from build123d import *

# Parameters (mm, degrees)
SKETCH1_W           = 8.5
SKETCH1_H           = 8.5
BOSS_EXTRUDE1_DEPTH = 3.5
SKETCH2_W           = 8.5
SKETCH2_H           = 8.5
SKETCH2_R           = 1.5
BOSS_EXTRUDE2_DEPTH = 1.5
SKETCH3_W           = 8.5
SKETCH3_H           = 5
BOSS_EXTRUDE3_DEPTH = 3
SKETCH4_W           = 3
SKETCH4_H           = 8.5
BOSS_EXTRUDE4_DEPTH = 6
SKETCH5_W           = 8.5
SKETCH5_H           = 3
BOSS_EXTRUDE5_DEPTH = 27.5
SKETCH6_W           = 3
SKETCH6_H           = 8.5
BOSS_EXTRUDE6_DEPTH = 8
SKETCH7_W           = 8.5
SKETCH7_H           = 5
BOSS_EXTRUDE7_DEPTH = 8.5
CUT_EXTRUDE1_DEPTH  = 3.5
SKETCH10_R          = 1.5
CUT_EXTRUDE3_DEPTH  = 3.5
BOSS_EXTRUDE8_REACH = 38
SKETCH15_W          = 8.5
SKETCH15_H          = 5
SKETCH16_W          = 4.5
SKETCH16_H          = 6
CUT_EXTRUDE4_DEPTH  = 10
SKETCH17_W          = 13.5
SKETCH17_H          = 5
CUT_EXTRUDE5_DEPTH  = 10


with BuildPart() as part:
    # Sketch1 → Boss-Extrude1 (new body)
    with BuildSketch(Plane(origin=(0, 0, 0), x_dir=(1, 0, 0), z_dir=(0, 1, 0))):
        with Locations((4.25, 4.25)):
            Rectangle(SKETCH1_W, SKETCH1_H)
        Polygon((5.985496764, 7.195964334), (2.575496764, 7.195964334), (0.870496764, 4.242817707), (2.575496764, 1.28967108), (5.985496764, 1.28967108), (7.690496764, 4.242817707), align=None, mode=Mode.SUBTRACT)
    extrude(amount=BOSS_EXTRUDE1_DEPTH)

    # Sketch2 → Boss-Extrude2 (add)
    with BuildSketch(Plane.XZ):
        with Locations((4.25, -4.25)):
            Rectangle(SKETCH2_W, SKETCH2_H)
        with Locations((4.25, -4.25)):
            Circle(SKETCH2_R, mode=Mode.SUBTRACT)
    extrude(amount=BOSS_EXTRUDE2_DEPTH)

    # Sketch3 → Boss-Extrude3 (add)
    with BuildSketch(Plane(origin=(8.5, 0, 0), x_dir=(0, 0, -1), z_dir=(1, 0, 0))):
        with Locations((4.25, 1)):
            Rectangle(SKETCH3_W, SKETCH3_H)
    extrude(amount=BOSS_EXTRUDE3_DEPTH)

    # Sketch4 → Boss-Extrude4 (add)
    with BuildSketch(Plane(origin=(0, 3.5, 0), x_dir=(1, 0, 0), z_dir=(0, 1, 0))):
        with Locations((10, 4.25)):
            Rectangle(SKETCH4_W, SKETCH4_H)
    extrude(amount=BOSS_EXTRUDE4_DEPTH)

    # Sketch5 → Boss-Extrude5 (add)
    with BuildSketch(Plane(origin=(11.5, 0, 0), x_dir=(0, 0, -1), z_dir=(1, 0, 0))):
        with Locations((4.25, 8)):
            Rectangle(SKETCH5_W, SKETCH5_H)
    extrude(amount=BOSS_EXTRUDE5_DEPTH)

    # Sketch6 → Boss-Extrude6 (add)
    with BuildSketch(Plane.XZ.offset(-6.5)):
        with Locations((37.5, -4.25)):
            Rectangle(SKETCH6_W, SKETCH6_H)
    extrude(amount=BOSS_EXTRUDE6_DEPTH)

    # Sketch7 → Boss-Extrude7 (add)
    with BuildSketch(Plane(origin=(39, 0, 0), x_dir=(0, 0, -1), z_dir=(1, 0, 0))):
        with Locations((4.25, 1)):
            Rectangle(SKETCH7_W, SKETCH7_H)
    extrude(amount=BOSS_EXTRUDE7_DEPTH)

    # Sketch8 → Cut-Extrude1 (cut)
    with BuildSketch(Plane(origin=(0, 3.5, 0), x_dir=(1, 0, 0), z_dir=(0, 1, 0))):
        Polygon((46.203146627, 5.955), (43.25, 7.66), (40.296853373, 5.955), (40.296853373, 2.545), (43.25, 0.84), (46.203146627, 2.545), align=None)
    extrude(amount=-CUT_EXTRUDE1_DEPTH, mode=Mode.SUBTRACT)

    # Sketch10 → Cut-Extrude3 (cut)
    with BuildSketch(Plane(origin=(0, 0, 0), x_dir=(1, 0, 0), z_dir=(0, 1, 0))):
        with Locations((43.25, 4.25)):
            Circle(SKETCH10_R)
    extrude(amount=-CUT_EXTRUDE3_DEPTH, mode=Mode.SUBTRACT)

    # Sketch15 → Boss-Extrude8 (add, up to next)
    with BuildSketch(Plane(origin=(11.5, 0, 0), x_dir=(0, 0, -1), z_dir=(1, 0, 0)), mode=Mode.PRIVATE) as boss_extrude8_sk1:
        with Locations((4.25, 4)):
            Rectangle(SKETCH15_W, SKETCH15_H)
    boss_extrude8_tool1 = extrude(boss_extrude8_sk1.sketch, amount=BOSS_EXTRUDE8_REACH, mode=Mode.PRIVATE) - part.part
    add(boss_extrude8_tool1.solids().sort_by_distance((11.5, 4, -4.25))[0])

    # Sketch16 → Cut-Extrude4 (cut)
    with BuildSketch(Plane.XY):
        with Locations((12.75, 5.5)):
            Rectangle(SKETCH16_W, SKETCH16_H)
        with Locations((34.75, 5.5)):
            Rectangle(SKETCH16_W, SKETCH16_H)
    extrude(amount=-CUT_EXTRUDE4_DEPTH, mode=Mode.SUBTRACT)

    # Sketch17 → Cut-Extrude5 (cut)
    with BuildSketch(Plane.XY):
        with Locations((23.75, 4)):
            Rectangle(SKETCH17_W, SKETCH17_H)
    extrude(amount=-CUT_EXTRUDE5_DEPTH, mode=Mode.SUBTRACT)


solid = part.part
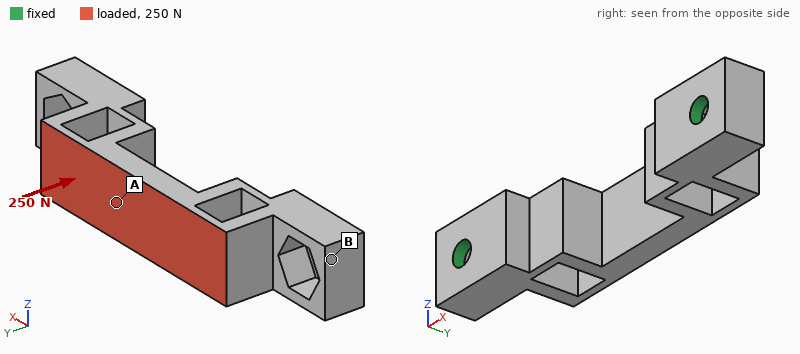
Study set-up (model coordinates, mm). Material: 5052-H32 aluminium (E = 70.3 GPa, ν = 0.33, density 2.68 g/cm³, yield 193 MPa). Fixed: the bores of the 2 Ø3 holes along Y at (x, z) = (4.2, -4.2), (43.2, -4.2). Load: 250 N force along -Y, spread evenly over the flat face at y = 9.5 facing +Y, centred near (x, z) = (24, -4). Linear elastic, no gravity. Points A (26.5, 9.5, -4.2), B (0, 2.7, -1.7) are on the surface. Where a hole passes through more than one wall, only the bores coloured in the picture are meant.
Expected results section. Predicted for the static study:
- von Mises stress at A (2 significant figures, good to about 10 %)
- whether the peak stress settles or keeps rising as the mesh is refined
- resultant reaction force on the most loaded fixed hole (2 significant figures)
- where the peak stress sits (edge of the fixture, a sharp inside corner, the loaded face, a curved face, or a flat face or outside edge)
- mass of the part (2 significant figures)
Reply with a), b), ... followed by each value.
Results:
a) 12 MPa
b) keeps rising
c) 170 N
d) edge of the fixture
e) 4.5 g
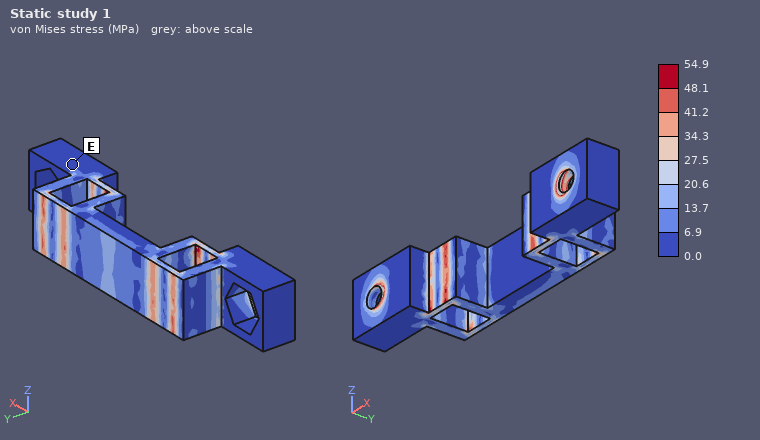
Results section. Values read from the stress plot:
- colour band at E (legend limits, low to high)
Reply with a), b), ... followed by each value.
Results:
a) 0.0 to 6.9 MPa
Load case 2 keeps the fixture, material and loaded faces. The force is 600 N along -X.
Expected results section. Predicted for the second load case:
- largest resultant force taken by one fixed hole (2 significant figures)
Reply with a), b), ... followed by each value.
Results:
a) 330 N
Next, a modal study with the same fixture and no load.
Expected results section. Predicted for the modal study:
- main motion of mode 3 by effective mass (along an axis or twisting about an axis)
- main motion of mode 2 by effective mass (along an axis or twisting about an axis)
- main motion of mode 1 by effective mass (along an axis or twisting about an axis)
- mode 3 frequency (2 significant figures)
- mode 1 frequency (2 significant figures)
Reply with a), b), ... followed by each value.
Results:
a) along X
b) along Y
c) along Z
d) 15 kHz
e) 8300 Hz
